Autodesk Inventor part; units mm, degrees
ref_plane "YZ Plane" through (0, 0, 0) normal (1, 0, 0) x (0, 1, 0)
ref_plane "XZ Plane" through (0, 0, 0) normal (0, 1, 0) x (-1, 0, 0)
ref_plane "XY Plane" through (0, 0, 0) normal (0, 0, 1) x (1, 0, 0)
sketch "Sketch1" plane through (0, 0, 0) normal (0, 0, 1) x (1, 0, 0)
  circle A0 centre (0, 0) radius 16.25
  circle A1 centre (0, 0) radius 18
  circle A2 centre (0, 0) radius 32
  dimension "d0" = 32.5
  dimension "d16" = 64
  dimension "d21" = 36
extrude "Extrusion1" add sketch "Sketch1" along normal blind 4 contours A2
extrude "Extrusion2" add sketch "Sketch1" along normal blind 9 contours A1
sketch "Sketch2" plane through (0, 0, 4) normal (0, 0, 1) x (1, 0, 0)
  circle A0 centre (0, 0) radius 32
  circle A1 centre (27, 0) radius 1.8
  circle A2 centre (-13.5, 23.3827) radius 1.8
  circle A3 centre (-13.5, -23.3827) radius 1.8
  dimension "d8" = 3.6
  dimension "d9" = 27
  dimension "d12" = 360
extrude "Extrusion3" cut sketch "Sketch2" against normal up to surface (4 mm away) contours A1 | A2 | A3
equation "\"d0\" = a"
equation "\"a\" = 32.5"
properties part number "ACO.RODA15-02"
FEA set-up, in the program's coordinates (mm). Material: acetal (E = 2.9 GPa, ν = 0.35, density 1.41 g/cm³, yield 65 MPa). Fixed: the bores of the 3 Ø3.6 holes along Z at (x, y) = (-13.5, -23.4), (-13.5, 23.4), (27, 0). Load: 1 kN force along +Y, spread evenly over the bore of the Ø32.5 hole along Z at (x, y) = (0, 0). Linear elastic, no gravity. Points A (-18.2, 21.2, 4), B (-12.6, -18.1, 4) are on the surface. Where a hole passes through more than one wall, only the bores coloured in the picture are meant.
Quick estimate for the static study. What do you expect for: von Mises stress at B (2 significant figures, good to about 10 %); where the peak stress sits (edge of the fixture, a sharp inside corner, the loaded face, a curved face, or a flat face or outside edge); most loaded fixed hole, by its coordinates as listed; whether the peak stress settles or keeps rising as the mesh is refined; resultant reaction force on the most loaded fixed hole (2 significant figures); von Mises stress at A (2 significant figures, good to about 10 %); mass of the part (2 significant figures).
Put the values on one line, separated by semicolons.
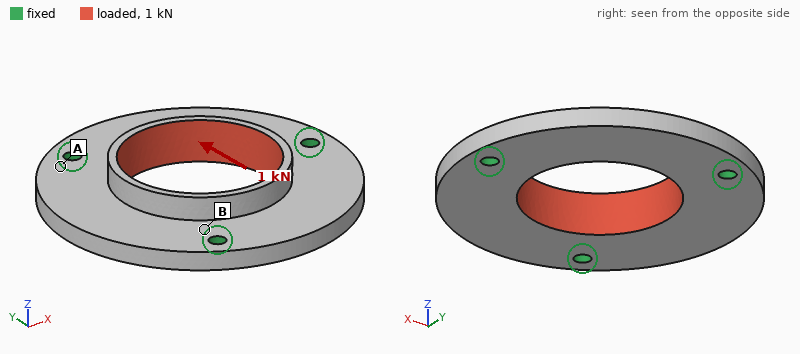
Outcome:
8.1 MPa; edge of the fixture; (27, 0); keeps rising; 420 N; 3.3 MPa; 15 g
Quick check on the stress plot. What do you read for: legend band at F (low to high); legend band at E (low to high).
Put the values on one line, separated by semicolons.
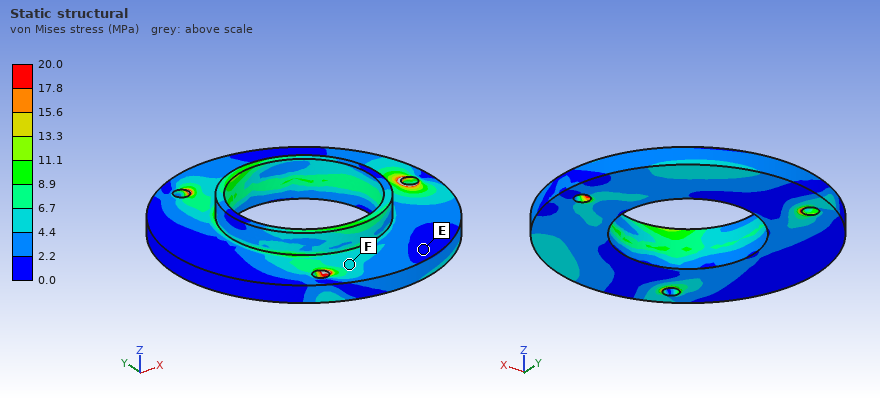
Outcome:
4.4 to 6.7 MPa; 0.0 to 2.2 MPa
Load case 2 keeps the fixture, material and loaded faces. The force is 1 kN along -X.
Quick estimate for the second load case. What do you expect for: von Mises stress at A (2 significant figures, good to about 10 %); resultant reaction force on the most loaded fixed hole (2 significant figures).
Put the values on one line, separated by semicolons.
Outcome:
9.2 MPa; 380 N
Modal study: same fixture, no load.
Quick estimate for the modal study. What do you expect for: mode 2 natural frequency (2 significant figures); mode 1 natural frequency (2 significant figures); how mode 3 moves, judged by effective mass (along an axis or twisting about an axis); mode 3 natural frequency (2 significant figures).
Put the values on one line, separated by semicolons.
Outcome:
1800 Hz; 1800 Hz; along Z; 2100 Hz
